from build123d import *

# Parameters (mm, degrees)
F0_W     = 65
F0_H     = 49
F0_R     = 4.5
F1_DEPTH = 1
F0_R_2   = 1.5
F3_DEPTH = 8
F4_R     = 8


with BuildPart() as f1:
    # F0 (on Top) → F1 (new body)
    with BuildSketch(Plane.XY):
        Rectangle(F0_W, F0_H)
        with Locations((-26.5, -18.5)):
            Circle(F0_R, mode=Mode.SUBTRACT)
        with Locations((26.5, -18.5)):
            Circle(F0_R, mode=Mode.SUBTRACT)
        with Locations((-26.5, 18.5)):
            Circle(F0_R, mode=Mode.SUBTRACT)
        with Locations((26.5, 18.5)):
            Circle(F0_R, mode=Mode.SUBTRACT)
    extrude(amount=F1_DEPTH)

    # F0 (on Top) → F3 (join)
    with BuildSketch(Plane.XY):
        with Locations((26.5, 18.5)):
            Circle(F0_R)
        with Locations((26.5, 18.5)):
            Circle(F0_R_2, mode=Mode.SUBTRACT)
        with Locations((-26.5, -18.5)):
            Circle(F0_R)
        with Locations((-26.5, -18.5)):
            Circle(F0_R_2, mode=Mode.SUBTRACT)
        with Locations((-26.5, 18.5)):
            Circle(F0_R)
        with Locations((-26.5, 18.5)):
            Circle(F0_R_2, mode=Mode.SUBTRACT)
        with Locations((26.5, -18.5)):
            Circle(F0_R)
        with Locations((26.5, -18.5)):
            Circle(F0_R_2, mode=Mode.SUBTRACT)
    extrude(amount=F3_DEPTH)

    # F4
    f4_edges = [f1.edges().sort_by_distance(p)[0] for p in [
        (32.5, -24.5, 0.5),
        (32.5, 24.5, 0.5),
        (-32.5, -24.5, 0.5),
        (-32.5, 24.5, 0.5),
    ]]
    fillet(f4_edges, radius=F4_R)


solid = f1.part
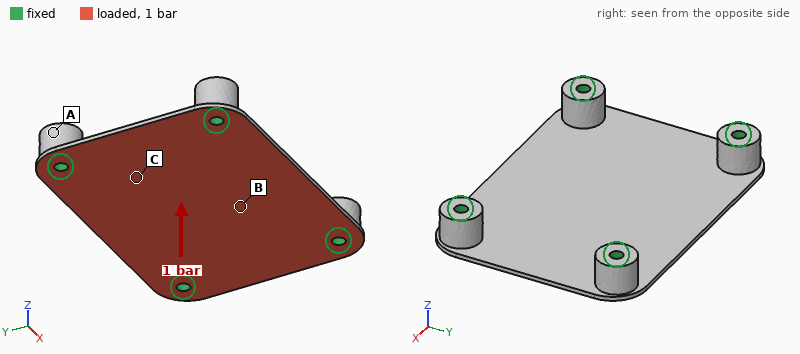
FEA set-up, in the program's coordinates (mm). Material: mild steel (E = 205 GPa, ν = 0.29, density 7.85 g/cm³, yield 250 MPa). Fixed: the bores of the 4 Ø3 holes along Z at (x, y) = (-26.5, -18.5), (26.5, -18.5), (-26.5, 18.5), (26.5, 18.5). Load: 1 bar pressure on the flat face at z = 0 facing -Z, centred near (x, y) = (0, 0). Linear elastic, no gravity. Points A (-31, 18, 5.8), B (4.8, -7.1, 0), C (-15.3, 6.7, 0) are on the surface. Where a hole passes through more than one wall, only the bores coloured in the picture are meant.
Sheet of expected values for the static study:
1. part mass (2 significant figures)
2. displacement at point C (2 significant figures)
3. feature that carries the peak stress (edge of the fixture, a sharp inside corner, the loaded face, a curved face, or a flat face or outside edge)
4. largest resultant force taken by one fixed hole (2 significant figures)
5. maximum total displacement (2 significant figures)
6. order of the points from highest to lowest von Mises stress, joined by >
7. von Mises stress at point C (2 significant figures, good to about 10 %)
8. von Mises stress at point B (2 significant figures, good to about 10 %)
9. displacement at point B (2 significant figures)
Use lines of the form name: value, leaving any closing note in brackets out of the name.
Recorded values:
part mass: 37 g
displacement at point C: 0.053 mm
feature that carries the peak stress: the loaded face
largest resultant force taken by one fixed hole: 86 N
maximum total displacement: 0.11 mm
order of the points from highest to lowest von Mises stress, joined by >: B > C > A
von Mises stress at point C: 25 MPa
von Mises stress at point B: 49 MPa
displacement at point B: 0.095 mm
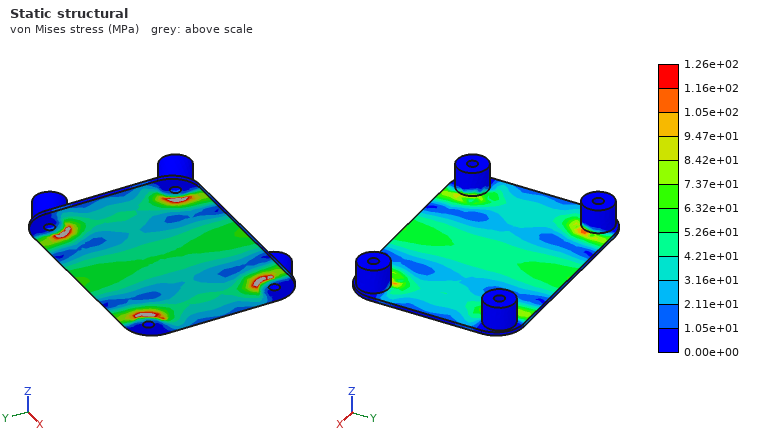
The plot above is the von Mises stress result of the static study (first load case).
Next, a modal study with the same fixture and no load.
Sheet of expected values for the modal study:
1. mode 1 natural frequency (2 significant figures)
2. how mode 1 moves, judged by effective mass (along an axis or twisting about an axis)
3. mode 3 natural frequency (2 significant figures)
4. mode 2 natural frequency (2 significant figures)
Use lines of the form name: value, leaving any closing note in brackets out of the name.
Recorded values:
mode 1 natural frequency: 2100 Hz
how mode 1 moves, judged by effective mass: along Z
mode 3 natural frequency: 4100 Hz
mode 2 natural frequency: 2900 Hz
